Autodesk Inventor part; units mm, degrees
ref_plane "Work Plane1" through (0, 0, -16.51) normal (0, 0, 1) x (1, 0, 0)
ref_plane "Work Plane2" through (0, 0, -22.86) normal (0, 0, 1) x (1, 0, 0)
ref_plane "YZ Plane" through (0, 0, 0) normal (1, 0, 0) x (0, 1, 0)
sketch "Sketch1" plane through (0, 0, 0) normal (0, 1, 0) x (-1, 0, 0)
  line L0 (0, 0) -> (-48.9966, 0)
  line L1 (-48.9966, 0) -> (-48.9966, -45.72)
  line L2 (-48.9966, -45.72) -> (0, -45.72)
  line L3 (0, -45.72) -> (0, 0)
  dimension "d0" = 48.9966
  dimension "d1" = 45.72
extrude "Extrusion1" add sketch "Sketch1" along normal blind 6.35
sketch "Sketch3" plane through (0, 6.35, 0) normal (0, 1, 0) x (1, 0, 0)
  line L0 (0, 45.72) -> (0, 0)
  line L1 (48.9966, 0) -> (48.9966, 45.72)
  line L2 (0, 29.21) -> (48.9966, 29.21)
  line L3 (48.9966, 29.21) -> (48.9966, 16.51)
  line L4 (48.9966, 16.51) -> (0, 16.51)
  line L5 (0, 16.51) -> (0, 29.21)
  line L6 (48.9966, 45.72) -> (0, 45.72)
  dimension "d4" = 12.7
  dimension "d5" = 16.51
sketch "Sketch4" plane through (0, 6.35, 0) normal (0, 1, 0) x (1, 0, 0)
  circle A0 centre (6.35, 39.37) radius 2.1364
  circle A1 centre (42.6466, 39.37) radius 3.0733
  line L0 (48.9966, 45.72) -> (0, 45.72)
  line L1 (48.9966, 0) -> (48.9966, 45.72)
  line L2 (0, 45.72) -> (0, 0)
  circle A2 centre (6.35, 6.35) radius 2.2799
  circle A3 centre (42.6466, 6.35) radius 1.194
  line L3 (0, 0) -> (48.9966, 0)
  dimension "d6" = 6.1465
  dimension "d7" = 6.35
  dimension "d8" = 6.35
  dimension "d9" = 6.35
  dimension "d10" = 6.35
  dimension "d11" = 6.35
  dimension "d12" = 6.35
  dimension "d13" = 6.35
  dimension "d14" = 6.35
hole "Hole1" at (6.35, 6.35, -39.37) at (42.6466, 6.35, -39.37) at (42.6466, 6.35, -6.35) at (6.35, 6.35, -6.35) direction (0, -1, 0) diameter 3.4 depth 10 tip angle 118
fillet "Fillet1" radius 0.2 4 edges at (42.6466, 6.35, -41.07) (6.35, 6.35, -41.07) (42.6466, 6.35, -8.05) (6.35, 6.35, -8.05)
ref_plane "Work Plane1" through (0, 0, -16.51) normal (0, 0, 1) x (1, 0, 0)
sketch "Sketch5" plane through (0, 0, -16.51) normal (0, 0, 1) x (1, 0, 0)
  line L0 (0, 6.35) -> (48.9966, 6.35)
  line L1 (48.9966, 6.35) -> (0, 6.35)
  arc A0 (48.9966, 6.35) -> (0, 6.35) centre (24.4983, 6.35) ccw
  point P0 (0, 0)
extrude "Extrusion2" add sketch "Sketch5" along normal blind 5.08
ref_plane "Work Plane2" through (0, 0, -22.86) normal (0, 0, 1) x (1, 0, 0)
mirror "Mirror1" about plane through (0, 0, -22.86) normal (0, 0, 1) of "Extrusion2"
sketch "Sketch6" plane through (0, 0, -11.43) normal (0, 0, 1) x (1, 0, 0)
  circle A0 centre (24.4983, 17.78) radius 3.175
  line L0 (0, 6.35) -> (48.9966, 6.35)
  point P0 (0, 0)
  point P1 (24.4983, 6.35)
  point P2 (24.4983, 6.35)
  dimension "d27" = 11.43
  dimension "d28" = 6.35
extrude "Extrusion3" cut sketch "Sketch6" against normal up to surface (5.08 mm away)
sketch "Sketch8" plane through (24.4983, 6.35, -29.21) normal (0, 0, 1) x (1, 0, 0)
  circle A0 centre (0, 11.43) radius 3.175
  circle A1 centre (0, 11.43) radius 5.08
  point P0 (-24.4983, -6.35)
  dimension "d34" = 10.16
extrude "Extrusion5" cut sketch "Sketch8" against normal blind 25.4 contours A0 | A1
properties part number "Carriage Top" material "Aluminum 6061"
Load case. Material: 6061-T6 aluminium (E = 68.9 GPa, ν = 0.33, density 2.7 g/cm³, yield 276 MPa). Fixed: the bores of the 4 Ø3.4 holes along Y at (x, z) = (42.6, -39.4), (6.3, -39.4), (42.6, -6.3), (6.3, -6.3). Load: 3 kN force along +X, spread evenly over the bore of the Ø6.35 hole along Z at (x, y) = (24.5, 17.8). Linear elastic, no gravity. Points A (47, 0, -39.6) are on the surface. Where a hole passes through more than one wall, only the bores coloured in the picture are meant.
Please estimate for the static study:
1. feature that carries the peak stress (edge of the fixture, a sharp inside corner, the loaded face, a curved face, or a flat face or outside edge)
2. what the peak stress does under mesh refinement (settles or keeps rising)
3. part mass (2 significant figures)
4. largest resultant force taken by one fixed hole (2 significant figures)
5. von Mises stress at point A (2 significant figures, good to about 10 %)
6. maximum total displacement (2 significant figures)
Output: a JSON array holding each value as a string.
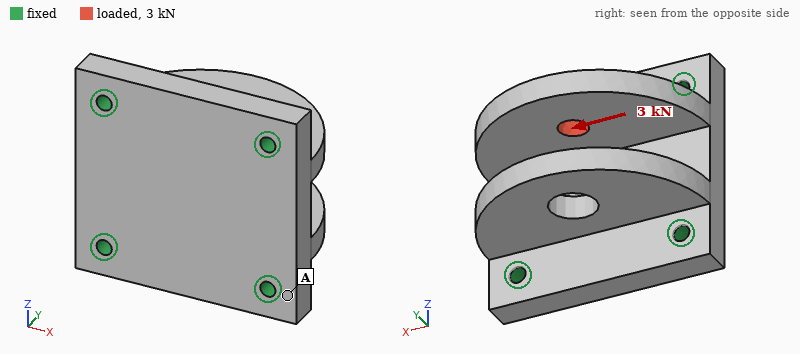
["edge of the fixture", "keeps rising", "62 g", "1.5 kN", "9.2 MPa", "21 µm"]
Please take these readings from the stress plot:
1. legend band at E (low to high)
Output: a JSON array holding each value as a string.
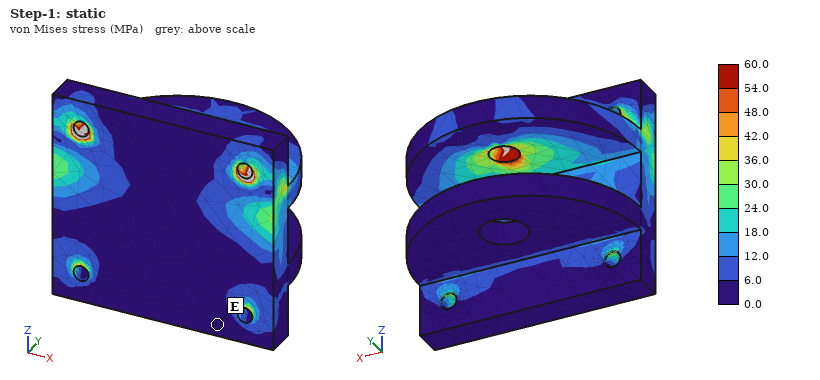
["0.0 to 6.0 MPa"]
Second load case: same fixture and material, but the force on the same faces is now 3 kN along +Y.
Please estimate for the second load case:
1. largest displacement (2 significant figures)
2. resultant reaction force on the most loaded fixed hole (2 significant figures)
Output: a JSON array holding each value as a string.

["19 µm", "1.2 kN"]
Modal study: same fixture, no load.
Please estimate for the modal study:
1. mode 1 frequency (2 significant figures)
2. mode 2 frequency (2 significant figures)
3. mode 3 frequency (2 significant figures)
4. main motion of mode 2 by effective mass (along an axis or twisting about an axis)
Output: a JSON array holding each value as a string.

["6600 Hz", "7400 Hz", "13 kHz", "along Z"]
